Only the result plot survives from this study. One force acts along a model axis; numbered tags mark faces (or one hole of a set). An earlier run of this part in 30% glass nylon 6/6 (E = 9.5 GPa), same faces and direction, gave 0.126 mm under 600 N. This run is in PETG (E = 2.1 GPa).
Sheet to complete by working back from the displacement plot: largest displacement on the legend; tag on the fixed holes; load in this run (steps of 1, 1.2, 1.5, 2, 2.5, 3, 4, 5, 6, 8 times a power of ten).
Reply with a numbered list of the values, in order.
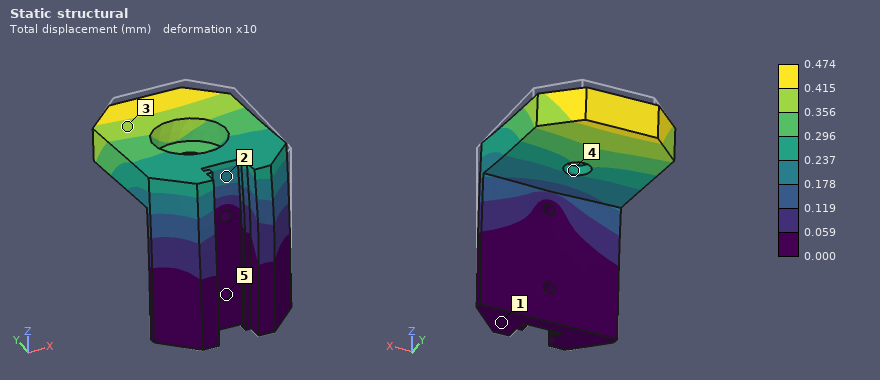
1. 0.474 mm
2. 5
3. 500 N
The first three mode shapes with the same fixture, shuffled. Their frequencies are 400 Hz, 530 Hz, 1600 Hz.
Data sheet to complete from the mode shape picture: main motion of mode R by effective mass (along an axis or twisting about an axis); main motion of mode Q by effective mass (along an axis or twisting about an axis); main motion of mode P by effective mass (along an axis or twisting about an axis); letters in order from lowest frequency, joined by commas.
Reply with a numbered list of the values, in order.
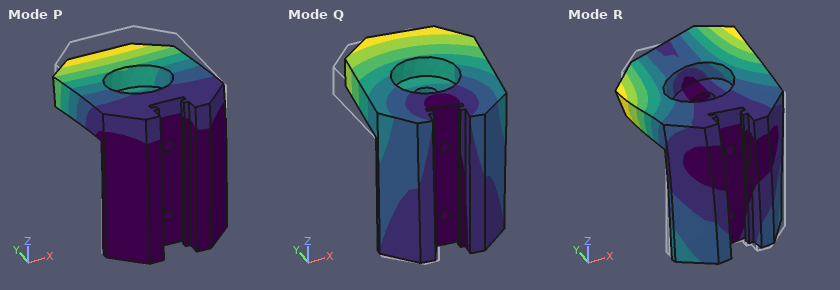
1. twisting about Y
2. along X
3. along Z
4. Q, P, R
